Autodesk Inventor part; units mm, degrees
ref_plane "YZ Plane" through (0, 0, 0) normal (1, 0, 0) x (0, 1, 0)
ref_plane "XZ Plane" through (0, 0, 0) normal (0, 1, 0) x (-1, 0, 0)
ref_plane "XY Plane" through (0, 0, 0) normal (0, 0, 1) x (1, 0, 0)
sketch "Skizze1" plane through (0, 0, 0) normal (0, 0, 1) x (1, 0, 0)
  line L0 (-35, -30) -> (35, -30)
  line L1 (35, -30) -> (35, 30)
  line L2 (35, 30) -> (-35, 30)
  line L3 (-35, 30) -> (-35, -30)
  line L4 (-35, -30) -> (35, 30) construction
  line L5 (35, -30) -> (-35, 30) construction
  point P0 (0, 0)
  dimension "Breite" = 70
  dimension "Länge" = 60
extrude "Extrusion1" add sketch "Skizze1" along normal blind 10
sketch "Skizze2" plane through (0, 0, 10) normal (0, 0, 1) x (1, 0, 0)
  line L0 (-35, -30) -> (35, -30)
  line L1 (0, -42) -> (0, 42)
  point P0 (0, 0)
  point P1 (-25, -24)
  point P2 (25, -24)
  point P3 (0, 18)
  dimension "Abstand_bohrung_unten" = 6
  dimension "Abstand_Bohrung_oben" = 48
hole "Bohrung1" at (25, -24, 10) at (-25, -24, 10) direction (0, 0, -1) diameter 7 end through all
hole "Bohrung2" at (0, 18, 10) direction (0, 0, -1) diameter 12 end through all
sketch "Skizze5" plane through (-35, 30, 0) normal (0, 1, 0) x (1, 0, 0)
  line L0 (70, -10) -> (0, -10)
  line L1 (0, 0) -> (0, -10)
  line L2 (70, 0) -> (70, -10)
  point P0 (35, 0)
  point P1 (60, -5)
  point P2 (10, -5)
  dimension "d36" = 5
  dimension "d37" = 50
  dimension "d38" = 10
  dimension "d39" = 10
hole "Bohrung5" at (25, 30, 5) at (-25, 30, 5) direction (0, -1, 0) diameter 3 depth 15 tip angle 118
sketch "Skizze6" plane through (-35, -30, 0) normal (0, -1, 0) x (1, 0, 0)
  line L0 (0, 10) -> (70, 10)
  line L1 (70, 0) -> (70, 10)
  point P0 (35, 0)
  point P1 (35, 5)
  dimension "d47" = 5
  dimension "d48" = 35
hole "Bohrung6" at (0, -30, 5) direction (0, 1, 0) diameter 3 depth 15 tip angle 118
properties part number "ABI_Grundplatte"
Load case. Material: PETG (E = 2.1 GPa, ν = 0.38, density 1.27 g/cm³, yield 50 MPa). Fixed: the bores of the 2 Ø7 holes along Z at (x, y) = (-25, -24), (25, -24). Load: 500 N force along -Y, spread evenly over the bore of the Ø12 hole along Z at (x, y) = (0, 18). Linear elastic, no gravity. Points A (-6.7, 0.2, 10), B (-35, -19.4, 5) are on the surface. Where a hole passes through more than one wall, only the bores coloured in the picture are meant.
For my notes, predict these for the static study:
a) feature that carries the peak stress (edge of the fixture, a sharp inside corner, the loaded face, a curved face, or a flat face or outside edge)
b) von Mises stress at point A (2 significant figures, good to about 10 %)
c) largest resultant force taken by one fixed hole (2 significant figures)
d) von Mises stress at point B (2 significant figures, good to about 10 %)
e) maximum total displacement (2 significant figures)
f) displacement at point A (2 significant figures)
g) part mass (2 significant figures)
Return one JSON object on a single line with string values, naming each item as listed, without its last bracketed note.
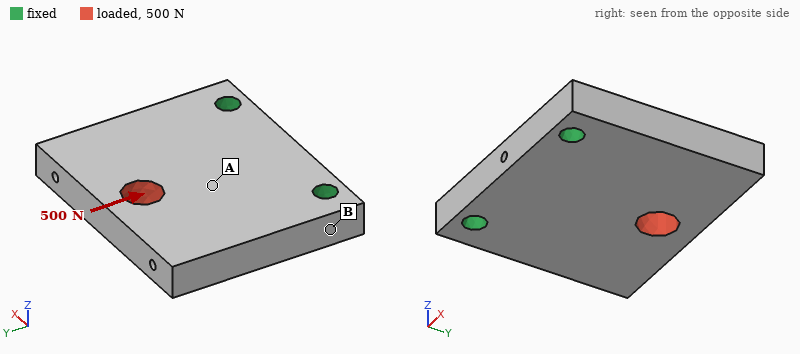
{"feature that carries the peak stress": "the loaded face", "von Mises stress at point A": "1.1 MPa", "largest resultant force taken by one fixed hole": "260 N", "von Mises stress at point B": "0.38 MPa", "maximum total displacement": "44 µm", "displacement at point A": "19 µm", "part mass": "51 g"}
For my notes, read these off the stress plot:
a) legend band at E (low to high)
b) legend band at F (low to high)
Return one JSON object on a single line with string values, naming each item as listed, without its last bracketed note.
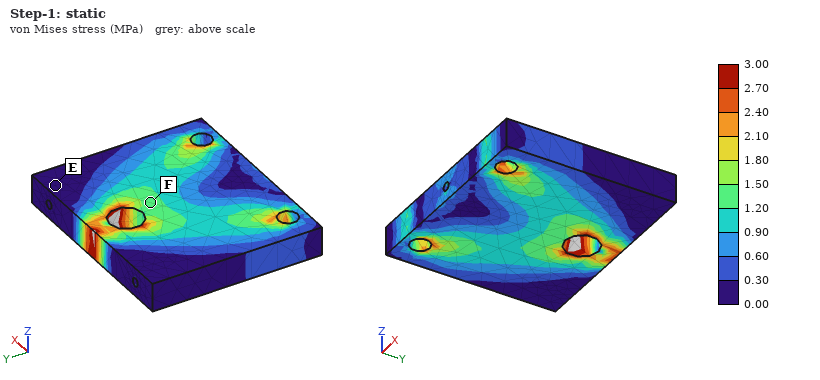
{"legend band at E": "0.00 to 0.30 MPa", "legend band at F": "1.20 to 1.50 MPa"}
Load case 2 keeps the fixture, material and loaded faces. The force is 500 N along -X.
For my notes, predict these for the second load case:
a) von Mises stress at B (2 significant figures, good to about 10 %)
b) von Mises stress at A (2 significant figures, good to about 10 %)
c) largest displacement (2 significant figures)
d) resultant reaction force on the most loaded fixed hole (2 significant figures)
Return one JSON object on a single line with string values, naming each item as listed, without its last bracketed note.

{"von Mises stress at B": "1.6 MPa", "von Mises stress at A": "1.9 MPa", "largest displacement": "95 µm", "resultant reaction force on the most loaded fixed hole": "460 N"}
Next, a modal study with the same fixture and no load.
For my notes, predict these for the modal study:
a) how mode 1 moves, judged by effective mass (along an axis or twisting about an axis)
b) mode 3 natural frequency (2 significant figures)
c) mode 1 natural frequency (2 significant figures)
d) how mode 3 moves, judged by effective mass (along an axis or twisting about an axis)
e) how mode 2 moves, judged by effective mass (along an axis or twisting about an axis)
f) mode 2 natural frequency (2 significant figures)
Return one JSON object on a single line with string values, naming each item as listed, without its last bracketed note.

{"how mode 1 moves, judged by effective mass": "along Z", "mode 3 natural frequency": "2600 Hz", "mode 1 natural frequency": "650 Hz", "how mode 3 moves, judged by effective mass": "along X", "how mode 2 moves, judged by effective mass": "twisting about Y", "mode 2 natural frequency": "1300 Hz"}
